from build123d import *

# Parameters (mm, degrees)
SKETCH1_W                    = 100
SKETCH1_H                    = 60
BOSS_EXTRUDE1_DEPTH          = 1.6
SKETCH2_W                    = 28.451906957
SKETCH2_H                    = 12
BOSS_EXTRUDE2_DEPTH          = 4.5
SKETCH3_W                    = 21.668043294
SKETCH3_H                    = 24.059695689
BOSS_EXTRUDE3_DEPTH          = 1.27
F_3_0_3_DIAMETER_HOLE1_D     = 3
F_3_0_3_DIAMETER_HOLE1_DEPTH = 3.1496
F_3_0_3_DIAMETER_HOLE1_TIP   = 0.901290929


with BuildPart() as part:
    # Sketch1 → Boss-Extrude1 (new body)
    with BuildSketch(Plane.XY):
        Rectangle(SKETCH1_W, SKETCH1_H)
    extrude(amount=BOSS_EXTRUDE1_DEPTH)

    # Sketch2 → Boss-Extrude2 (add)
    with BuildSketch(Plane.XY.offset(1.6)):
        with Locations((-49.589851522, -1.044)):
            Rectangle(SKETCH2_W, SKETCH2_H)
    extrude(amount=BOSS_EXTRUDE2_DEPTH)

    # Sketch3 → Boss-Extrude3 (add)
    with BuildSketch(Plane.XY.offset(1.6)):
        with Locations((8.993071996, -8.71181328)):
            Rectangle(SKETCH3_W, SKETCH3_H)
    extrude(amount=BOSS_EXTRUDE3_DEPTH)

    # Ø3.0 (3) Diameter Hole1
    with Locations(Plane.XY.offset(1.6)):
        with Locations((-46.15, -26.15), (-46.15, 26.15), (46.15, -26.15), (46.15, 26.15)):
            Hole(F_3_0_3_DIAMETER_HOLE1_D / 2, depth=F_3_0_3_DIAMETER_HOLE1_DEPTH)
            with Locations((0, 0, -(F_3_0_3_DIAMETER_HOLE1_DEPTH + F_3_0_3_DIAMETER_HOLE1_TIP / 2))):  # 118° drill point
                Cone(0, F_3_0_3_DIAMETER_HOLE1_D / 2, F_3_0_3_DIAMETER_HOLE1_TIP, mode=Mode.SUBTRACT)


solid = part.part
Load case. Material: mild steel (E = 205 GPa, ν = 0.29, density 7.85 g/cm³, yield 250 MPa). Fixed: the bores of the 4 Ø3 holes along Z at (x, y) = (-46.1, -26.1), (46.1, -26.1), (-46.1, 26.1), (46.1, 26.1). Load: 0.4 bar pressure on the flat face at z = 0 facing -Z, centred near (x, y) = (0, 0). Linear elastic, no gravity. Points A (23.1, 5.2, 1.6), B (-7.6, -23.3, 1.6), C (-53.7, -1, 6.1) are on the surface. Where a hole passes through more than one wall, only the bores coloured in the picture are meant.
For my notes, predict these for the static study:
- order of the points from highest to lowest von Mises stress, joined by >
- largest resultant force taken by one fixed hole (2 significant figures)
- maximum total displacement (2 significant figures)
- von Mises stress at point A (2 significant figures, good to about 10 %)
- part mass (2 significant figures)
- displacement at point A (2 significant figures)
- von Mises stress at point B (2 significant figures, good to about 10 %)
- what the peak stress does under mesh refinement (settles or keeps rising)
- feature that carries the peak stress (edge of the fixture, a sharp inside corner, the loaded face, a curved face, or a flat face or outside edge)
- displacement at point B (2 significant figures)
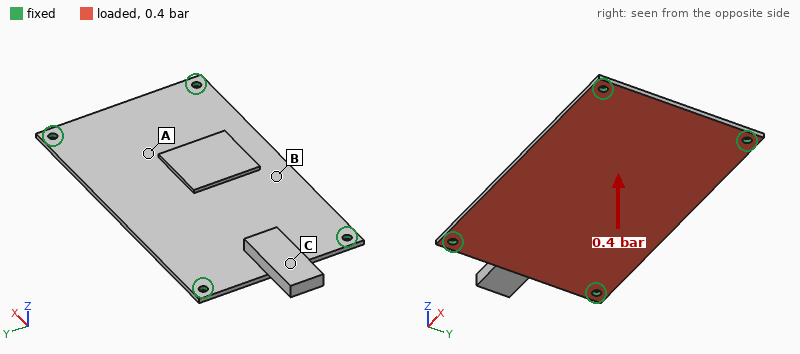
B > A > C
72 N
0.14 mm
24 MPa
92 g
0.091 mm
41 MPa
keeps rising
edge of the fixture
0.12 mm
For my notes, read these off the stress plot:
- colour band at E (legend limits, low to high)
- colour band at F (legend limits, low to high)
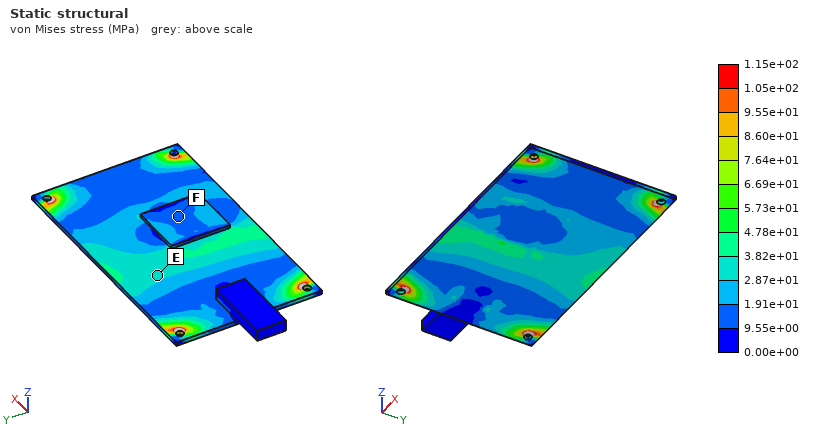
2.87e+01 to 3.82e+01 MPa
9.55e+00 to 1.91e+01 MPa
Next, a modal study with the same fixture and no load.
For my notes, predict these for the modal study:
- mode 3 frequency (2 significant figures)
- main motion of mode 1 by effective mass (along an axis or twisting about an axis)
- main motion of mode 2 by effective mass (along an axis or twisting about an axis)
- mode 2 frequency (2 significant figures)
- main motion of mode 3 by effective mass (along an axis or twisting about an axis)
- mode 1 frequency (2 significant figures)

1800 Hz
along Z
twisting about X
1500 Hz
along Z
830 Hz
